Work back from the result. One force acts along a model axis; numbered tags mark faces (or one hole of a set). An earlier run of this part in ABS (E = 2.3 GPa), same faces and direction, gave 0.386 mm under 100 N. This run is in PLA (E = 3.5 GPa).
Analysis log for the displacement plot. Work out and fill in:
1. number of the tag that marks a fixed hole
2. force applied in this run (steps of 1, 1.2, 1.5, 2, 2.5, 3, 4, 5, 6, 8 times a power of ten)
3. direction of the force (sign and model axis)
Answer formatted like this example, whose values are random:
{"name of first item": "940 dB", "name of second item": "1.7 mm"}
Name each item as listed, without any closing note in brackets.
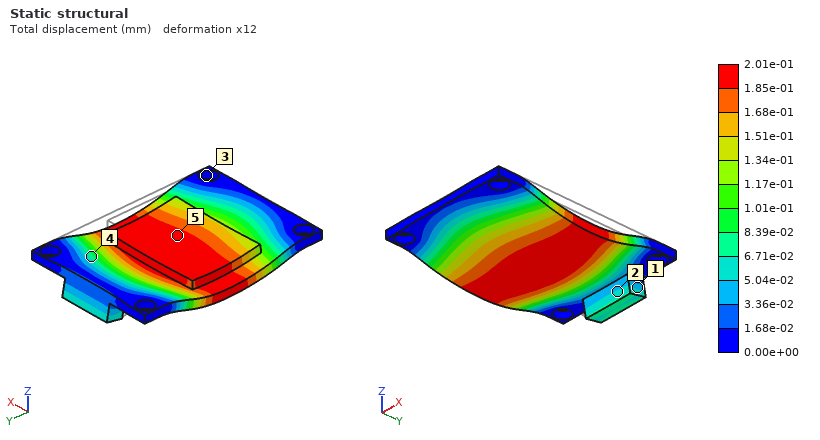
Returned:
{"number of the tag that marks a fixed hole": "3", "force applied in this run": "80 N", "direction of the force": "-Z"}
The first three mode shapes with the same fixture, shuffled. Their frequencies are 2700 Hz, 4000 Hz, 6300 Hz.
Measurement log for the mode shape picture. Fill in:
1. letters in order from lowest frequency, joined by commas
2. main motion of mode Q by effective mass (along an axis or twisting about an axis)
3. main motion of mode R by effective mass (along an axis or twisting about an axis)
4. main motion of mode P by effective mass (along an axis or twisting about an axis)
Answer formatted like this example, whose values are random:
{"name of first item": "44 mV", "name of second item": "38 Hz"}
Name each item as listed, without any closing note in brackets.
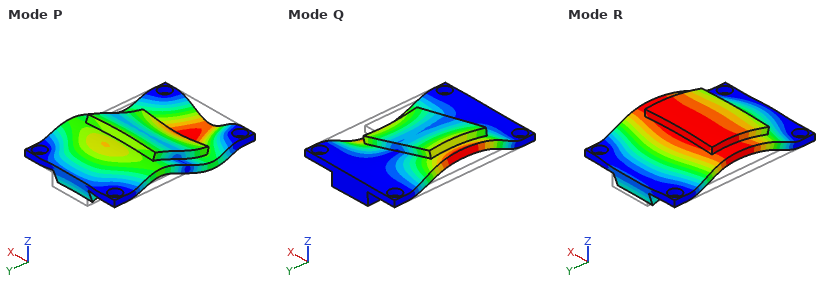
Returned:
{"letters in order from lowest frequency, joined by commas": "R, Q, P", "main motion of mode Q by effective mass": "twisting about Y", "main motion of mode R by effective mass": "along Z", "main motion of mode P by effective mass": "twisting about X"}
